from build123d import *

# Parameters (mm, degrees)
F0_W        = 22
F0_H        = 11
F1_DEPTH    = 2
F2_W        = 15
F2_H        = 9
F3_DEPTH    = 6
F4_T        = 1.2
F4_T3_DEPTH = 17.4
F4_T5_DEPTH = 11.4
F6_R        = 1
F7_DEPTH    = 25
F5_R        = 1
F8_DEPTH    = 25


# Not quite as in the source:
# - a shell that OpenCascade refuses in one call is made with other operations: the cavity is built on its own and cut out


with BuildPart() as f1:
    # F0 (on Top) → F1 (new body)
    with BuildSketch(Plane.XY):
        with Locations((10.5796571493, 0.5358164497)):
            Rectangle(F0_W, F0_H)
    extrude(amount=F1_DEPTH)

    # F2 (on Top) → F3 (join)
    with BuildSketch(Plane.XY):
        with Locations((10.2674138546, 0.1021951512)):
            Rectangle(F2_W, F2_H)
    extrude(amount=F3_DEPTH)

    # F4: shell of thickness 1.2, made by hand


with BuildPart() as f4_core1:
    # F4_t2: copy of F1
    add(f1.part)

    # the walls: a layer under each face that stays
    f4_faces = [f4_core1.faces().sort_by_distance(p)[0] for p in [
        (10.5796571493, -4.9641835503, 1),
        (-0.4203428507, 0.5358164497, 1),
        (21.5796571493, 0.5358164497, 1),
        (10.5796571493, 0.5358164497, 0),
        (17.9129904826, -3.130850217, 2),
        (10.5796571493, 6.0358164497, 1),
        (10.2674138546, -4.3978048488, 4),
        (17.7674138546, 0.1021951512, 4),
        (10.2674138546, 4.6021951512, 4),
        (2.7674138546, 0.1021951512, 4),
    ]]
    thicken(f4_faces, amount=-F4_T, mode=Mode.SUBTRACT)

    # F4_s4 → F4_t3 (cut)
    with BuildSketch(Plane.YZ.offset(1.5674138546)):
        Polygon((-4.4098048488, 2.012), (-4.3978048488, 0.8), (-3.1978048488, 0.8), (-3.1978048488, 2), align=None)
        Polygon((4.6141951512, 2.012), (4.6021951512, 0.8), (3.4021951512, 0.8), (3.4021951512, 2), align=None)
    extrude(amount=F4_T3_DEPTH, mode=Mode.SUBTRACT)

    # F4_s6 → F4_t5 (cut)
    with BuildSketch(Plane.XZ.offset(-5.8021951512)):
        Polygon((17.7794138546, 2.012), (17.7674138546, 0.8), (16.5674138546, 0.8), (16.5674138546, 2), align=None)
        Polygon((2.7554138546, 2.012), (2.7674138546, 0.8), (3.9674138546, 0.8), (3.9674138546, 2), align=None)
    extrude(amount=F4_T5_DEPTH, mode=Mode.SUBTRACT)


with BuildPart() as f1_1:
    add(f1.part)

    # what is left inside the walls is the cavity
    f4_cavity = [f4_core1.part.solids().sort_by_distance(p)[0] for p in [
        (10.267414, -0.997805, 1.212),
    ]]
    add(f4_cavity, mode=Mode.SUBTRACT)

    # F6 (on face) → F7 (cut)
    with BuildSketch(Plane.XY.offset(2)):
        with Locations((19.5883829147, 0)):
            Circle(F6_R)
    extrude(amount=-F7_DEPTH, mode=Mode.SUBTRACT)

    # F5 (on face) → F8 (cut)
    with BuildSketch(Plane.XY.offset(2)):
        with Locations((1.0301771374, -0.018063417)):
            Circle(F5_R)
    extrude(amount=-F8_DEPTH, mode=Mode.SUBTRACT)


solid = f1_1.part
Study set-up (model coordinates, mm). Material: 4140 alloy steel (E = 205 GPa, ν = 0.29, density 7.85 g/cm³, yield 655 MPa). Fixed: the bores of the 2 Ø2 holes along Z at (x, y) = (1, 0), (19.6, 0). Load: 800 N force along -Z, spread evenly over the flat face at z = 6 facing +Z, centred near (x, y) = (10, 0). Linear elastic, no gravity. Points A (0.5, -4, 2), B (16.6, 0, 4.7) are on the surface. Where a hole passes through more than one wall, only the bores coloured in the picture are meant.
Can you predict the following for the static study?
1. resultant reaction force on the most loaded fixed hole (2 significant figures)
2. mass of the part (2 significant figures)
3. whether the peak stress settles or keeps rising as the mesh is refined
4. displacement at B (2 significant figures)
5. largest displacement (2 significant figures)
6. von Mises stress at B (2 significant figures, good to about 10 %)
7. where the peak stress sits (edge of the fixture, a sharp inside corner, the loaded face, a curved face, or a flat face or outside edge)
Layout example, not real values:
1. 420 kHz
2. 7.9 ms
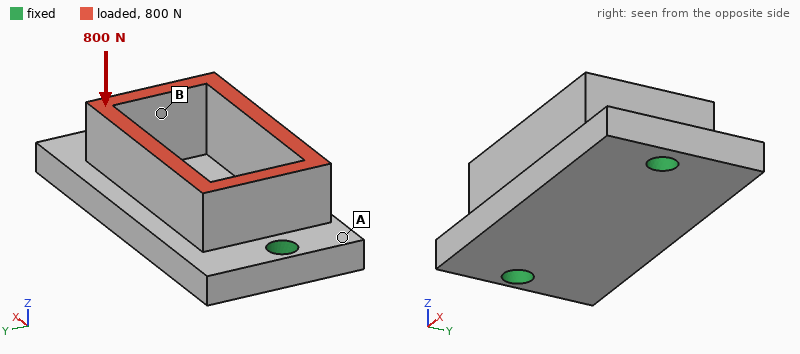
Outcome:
1. 410 N
2. 4.8 g
3. keeps rising
4. 2.9 µm
5. 5.4 µm
6. 50 MPa
7. edge of the fixture
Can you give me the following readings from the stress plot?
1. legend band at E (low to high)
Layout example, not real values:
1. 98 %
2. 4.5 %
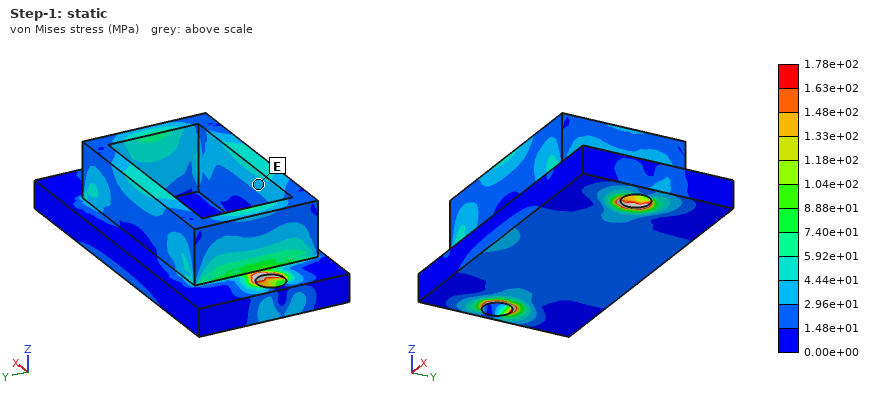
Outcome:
1. 2.96e+01 to 4.44e+01 MPa
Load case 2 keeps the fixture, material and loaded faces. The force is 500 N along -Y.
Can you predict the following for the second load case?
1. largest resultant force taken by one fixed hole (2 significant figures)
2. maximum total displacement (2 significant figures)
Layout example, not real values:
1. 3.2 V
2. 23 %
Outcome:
1. 250 N
2. 23 µm
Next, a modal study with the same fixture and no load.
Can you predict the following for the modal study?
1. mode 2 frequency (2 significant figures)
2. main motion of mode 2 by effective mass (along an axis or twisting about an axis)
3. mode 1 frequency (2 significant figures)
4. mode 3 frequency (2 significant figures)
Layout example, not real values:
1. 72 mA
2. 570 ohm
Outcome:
1. 35 kHz
2. along Z
3. 23 kHz
4. 40 kHz
